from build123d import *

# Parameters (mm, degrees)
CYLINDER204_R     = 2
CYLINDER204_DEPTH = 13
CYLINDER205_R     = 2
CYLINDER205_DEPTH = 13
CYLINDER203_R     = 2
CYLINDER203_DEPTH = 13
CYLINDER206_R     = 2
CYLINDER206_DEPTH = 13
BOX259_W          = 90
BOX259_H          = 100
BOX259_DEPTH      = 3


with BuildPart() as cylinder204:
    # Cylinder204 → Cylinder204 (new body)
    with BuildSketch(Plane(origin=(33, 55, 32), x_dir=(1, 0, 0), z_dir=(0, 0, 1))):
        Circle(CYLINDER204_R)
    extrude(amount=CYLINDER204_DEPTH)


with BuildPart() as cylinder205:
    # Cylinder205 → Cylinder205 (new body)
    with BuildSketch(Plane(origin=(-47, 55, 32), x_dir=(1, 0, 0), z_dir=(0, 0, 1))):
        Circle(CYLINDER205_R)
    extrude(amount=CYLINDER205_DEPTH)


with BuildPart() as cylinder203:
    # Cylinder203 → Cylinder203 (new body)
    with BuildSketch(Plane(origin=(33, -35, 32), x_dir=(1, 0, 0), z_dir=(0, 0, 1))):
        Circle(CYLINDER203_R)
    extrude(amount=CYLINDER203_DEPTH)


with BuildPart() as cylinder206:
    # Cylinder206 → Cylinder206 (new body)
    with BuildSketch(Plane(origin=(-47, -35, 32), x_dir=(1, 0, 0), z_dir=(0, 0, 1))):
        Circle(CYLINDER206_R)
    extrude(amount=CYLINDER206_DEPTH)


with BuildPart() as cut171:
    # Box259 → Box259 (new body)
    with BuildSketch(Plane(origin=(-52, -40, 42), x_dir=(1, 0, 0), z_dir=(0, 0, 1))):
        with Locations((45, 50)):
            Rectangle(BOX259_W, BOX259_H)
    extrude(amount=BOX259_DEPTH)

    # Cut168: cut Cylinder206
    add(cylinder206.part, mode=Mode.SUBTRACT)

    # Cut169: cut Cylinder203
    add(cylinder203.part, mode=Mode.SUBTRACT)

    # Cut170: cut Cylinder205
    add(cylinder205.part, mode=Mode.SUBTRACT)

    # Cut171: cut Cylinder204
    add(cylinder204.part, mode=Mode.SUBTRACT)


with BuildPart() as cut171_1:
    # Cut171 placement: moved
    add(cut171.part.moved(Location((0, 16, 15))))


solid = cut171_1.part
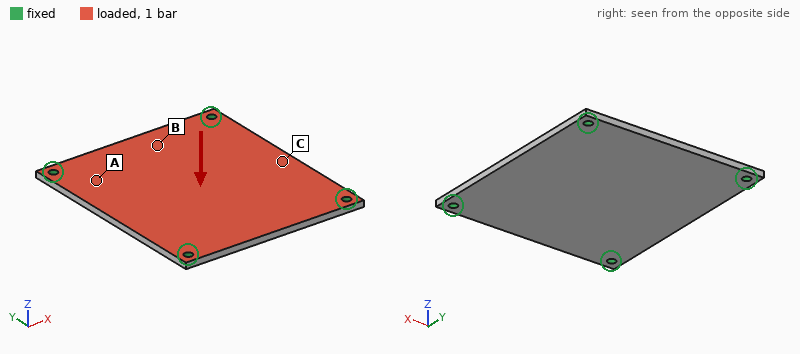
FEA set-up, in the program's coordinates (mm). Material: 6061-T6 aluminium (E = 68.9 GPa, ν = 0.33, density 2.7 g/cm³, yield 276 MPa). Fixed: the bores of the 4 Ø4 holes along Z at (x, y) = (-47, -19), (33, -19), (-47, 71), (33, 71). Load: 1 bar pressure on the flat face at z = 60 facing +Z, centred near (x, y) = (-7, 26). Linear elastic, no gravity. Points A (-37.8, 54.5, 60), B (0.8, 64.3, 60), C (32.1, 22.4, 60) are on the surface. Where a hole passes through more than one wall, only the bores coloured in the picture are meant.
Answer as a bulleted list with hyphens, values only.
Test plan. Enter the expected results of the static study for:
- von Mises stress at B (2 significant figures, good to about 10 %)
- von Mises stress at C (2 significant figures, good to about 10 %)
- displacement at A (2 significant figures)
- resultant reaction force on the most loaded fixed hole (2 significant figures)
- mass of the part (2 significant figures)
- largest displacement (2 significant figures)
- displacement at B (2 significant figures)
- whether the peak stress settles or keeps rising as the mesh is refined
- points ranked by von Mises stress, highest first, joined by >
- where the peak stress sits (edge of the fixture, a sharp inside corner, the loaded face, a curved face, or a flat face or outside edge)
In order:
- 23 MPa
- 32 MPa
- 0.100 mm
- 220 N
- 72 g
- 0.25 mm
- 0.13 mm
- keeps rising
- C > B > A
- edge of the fixture
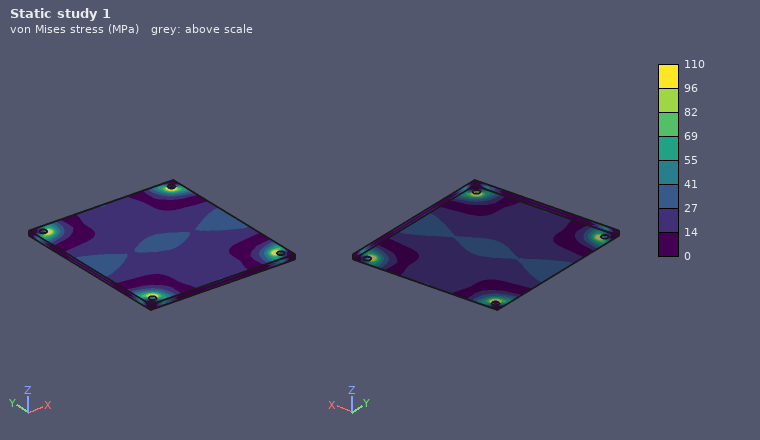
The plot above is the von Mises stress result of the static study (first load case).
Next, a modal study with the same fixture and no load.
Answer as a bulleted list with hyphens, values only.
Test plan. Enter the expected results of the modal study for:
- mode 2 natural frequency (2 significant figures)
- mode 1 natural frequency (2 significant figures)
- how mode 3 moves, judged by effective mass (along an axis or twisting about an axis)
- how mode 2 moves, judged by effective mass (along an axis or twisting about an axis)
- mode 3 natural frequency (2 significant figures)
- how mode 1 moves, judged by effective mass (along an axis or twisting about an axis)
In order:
- 2200 Hz
- 1300 Hz
- twisting about X
- twisting about Y
- 2500 Hz
- along Z
